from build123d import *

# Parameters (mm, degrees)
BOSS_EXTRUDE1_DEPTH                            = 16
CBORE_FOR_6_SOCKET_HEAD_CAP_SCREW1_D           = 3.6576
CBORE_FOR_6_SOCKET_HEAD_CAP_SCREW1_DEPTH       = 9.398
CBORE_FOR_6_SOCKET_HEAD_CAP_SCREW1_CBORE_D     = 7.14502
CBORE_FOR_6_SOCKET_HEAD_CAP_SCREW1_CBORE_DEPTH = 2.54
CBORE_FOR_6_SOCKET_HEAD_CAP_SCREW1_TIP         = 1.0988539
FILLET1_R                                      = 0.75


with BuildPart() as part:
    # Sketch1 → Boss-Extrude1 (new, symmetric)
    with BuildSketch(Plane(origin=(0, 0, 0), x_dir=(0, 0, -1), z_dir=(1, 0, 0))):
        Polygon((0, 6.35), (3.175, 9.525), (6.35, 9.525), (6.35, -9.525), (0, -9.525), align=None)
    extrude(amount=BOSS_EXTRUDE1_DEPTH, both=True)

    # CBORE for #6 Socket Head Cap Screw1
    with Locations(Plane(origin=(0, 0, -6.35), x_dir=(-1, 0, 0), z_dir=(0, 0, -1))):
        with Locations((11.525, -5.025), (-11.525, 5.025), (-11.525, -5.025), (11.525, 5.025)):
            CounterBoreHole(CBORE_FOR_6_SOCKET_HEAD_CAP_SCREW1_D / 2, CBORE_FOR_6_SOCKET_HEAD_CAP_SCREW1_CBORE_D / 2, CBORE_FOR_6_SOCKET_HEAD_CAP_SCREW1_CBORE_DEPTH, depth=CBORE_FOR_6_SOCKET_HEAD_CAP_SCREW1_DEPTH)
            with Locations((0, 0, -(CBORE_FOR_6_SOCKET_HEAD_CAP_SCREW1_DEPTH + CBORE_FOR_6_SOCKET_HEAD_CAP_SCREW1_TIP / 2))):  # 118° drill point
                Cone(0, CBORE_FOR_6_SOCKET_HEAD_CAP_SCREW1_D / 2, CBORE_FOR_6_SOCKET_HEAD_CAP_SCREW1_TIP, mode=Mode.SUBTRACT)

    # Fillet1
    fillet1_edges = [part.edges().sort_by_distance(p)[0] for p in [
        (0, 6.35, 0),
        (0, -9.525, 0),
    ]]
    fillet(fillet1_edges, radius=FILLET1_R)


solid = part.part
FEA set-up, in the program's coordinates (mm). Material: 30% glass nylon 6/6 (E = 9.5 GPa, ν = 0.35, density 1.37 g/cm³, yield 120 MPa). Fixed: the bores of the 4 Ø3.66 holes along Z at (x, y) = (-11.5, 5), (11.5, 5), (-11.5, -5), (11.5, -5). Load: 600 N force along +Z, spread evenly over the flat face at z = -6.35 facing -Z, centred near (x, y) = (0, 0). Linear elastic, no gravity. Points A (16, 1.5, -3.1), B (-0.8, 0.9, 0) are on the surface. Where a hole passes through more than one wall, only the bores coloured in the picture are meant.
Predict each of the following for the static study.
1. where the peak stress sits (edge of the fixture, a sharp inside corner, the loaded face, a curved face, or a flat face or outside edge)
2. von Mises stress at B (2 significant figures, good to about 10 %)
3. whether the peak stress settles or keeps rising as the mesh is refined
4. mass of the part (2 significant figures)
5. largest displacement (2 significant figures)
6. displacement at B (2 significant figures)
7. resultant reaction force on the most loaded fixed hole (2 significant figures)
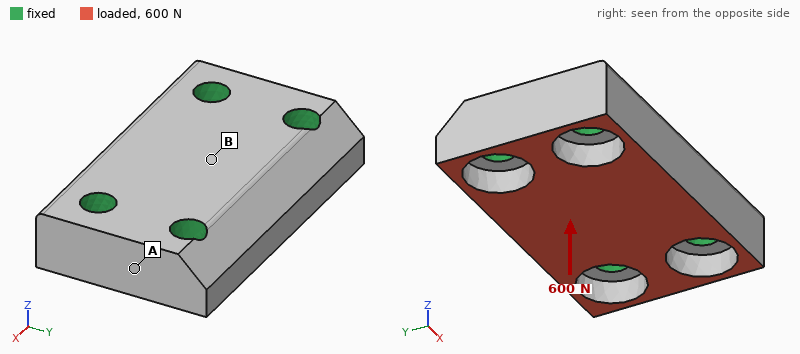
edge of the fixture
4.4 MPa
keeps rising
4.3 g
14 µm
10 µm
160 N
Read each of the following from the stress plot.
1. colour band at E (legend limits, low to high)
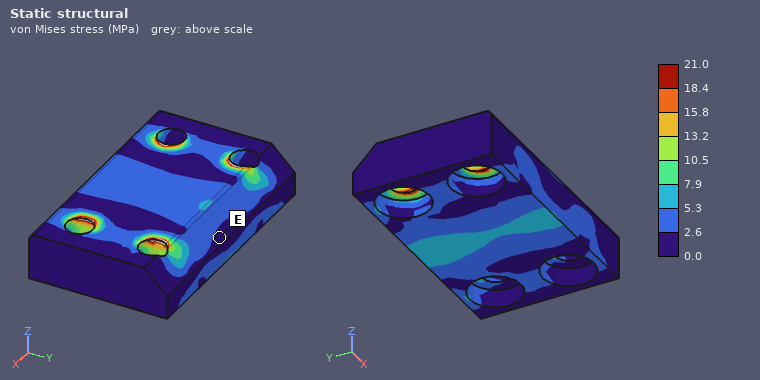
0.0 to 2.6 MPa
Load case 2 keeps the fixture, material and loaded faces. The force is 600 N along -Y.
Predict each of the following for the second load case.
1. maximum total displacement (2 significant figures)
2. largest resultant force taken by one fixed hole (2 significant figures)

18 µm
200 N
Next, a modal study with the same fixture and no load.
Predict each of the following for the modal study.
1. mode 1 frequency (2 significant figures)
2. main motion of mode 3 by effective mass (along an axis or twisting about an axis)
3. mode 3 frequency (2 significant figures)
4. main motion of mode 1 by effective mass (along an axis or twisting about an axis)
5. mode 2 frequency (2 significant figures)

21 kHz
along Y
30 kHz
along Z
23 kHz
